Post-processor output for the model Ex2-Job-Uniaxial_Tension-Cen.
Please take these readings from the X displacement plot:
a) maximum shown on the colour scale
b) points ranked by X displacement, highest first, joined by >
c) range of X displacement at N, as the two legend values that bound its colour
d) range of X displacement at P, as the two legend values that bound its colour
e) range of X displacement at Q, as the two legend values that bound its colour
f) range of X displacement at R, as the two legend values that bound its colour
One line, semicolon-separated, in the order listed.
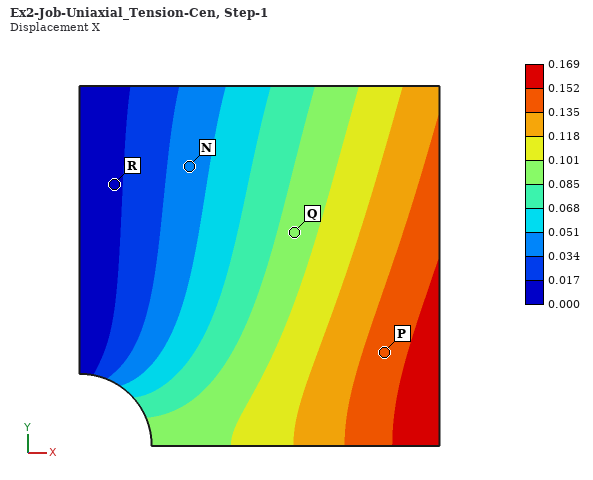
0.169; P > Q > N > R; 0.034 to 0.051; 0.135 to 0.152; 0.085 to 0.101; 0.000 to 0.017
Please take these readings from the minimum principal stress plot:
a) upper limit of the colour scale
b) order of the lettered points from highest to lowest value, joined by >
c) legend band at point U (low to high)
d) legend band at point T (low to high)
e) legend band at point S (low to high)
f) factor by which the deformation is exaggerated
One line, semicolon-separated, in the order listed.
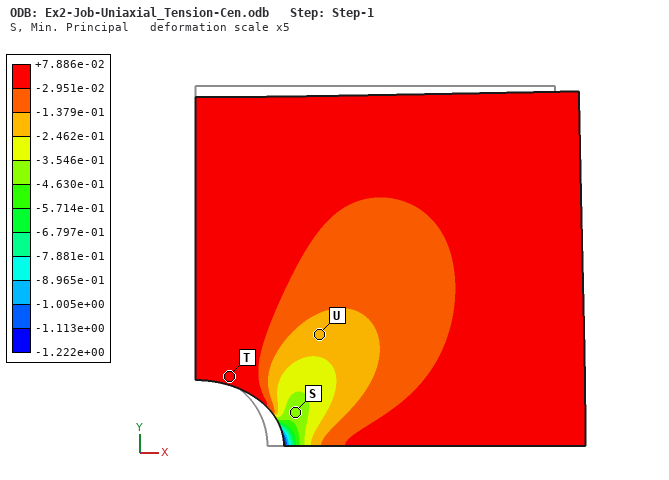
+7.886e-02; T > U > S; -2.462e-01 to -1.379e-01; -2.951e-02 to +7.886e-02; -4.630e-01 to -3.546e-01; 5
